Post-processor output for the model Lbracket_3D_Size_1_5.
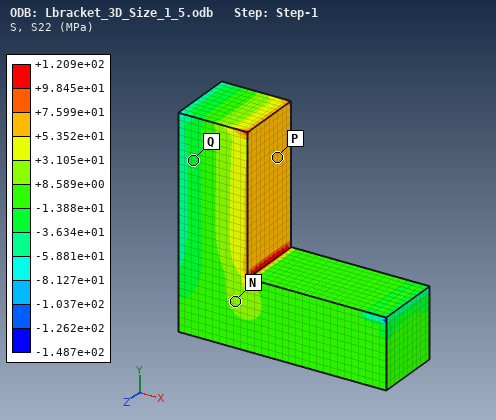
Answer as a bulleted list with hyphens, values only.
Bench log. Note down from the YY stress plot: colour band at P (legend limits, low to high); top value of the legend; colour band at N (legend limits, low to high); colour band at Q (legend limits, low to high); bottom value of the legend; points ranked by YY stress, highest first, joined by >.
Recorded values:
- +5.352e+01 to +7.599e+01 MPa
- +1.209e+02 MPa
- +8.589e+00 to +3.105e+01 MPa
- -3.634e+01 to -1.388e+01 MPa
- -1.487e+02 MPa
- P > N > Q
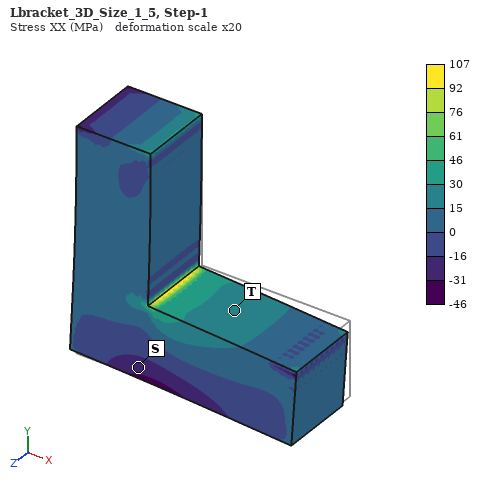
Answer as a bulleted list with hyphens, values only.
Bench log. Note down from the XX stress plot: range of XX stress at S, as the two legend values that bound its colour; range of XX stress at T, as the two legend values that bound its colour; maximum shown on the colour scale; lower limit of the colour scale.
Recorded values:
- -31 to -16 MPa
- 15 to 30 MPa
- 107 MPa
- -46 MPa
